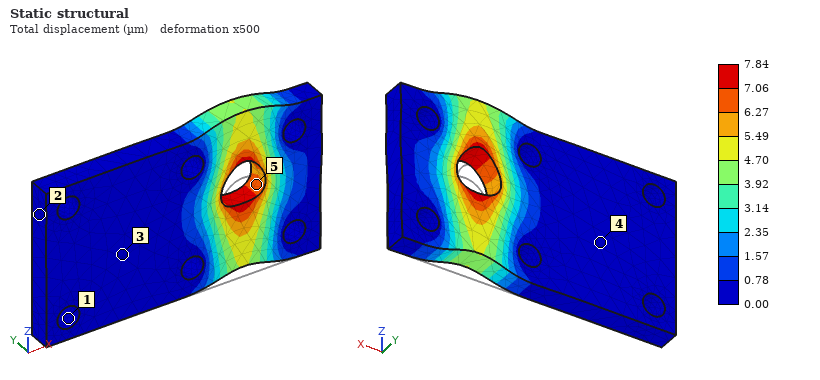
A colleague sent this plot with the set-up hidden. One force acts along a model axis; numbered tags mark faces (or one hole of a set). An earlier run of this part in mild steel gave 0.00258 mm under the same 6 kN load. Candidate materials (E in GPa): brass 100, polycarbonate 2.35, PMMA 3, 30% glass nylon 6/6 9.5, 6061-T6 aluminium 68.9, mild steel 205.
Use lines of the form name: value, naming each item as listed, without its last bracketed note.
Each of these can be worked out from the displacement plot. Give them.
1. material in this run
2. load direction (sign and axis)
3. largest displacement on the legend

material in this run: 6061-T6 aluminium
load direction: +Z
largest displacement on the legend: 7.84 µm
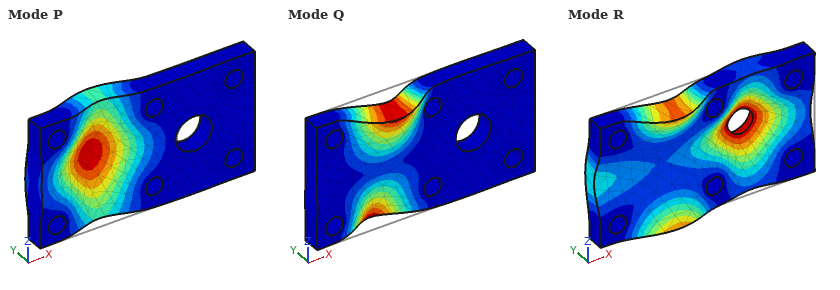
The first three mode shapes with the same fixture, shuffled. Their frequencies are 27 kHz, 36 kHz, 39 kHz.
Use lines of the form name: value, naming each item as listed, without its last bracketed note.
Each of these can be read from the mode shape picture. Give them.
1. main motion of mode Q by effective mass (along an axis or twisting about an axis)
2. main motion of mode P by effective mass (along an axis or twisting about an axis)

main motion of mode Q by effective mass: twisting about X
main motion of mode P by effective mass: along Y
